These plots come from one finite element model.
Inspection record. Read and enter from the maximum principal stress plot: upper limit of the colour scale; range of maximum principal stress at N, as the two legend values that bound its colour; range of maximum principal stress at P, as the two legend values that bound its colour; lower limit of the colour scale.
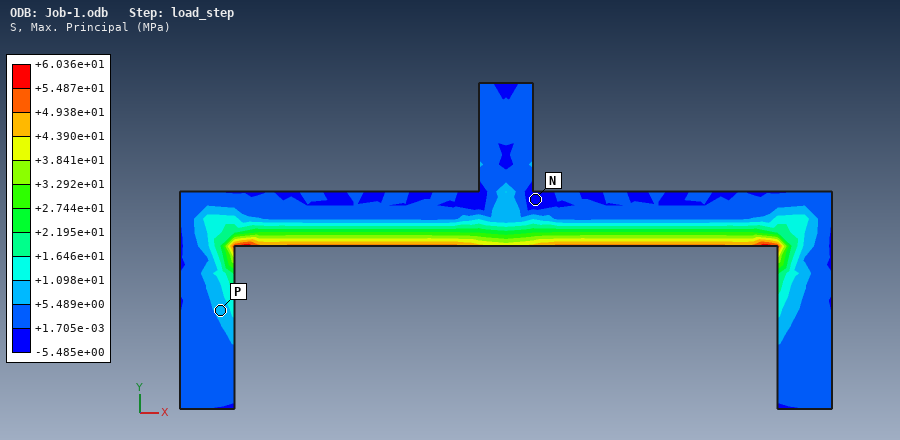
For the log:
+6.036e+01 MPa
-5.485e+00 to +1.705e-03 MPa
+5.489e+00 to +1.098e+01 MPa
-5.485e+00 MPa
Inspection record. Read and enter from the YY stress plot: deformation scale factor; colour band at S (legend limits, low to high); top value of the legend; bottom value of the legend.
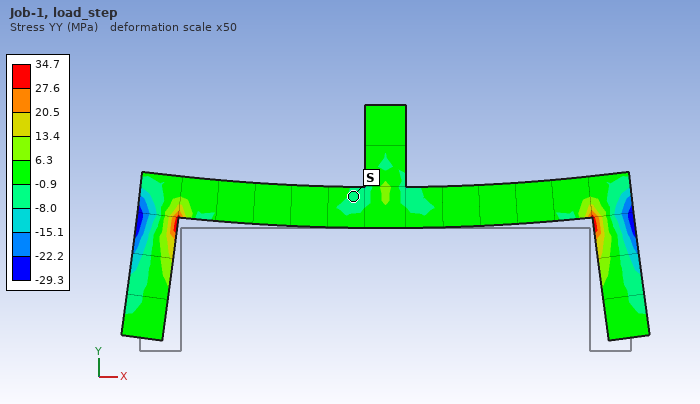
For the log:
50
-8.0 to -0.9 MPa
34.7 MPa
-29.3 MPa
